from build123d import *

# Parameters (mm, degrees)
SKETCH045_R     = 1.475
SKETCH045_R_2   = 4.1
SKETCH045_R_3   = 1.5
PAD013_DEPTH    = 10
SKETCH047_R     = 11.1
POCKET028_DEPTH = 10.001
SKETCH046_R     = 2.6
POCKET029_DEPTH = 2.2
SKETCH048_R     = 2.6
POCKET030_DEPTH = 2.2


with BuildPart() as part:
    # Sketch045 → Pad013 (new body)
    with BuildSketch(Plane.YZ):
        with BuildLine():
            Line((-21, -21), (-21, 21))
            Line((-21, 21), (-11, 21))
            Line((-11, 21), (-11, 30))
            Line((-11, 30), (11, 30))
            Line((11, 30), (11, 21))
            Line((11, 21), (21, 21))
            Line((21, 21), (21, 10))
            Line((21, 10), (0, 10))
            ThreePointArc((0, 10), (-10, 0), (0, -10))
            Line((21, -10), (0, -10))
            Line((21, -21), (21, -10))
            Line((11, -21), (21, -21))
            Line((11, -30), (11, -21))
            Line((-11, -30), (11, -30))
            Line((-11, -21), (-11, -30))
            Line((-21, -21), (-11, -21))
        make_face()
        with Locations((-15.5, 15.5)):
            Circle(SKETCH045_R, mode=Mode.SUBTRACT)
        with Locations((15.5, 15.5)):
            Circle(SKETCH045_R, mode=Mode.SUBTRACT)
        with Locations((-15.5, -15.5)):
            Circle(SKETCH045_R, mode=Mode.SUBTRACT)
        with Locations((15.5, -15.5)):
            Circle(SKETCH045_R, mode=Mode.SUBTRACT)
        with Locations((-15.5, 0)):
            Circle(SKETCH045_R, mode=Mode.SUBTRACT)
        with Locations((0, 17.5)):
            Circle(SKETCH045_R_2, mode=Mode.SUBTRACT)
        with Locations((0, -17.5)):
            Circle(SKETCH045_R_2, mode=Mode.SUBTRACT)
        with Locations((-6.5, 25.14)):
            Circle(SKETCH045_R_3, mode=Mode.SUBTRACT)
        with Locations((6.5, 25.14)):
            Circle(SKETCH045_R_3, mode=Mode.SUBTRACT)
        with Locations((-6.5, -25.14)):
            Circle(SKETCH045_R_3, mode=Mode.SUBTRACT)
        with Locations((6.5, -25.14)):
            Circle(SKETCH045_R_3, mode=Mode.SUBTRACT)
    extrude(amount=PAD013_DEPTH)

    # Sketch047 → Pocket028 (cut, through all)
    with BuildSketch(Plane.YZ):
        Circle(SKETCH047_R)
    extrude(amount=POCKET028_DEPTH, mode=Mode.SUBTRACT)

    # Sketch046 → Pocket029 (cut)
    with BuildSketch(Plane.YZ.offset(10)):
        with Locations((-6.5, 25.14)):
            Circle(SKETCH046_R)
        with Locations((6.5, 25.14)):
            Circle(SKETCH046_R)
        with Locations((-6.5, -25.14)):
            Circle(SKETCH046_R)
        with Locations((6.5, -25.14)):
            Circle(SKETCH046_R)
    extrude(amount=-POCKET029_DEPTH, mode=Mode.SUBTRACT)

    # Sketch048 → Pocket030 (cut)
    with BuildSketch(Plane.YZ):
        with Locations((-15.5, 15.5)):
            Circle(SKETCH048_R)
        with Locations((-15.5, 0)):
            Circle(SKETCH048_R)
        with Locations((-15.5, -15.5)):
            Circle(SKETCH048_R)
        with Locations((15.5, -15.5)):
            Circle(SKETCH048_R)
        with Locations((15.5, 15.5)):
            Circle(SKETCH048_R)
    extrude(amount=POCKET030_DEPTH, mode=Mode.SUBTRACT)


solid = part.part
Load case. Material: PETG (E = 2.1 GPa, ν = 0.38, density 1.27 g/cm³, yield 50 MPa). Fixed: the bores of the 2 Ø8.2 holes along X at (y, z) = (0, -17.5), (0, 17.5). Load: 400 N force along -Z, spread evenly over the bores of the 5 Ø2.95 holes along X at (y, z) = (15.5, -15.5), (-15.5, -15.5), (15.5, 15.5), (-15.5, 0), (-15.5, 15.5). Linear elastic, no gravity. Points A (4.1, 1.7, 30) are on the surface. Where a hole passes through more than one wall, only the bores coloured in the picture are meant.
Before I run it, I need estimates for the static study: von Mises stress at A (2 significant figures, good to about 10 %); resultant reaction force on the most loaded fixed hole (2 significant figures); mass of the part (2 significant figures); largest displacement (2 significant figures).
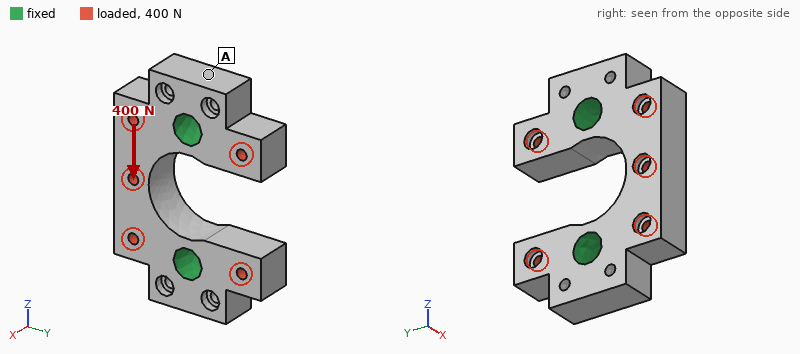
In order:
1.2 MPa
210 N
17 g
46 µm
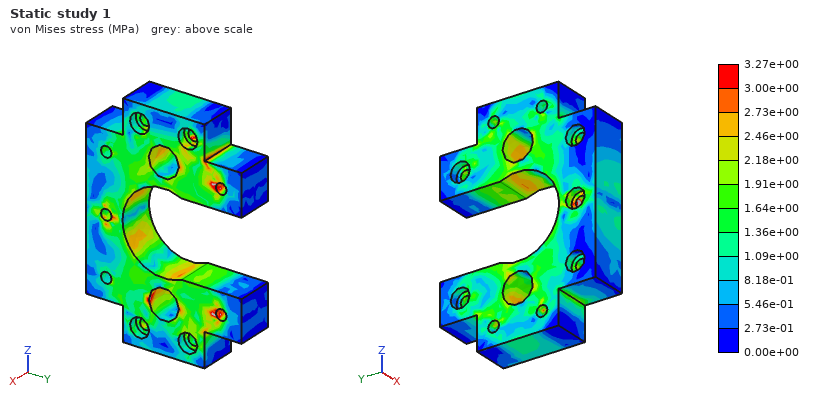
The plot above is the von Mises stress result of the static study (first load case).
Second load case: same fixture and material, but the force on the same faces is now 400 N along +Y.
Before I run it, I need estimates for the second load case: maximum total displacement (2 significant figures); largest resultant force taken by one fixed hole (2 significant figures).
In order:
19 µm
200 N
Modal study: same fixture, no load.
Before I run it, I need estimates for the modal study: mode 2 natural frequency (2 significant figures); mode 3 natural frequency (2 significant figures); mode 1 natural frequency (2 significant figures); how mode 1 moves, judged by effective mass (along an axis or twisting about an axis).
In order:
5700 Hz
5700 Hz
4000 Hz
along X
